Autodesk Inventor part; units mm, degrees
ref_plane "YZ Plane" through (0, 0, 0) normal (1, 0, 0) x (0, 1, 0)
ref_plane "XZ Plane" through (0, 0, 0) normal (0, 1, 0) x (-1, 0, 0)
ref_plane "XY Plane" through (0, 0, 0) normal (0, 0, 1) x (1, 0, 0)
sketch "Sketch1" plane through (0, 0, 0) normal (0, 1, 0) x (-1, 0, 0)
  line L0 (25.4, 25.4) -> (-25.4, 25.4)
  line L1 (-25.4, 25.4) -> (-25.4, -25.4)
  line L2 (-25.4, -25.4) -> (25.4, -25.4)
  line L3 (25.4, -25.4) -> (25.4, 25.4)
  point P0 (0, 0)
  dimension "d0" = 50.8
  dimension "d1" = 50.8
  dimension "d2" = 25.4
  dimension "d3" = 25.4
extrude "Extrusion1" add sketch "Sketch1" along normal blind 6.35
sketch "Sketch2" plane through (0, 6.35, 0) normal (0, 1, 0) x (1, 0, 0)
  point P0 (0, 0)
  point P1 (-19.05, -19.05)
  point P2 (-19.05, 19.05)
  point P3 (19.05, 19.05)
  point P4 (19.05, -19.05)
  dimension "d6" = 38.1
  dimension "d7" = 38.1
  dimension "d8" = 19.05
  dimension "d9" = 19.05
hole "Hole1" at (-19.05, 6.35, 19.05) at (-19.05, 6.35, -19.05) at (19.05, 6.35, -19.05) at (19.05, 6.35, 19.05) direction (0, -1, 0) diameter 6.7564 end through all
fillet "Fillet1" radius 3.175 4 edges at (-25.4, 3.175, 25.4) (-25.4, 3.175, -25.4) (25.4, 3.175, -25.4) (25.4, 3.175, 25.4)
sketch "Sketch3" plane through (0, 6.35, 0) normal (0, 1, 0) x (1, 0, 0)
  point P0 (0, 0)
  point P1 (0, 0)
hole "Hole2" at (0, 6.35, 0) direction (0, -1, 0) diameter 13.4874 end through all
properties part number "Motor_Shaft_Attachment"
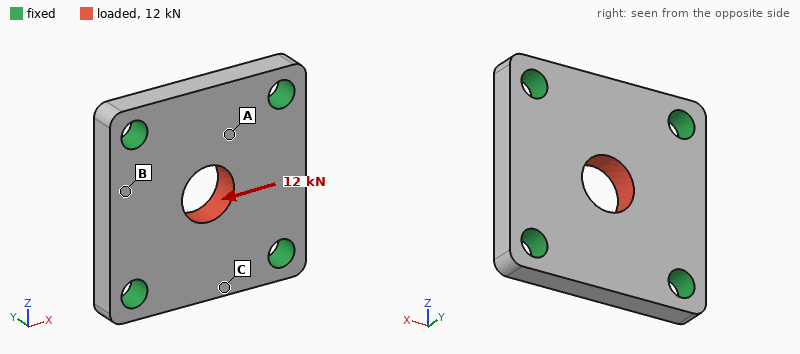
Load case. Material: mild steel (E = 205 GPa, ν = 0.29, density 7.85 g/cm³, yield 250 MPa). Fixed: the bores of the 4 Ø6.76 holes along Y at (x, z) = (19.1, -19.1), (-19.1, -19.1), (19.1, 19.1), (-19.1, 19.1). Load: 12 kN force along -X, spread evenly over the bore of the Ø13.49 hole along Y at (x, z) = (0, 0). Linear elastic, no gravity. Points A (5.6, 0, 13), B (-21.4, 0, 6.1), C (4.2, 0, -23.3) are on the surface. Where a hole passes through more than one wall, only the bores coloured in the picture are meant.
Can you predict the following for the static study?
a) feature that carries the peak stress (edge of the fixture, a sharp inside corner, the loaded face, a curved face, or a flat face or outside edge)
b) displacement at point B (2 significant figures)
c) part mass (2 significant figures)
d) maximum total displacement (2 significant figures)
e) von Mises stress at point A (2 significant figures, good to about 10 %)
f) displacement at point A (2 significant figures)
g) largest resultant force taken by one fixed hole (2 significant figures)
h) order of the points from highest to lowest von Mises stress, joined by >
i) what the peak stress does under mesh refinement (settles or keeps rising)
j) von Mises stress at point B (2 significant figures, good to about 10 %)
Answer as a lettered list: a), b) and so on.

a) edge of the fixture
b) 2.9 µm
c) 110 g
d) 5.1 µm
e) 32 MPa
f) 2.0 µm
g) 3.3 kN
h) A > B > C
i) keeps rising
j) 16 MPa
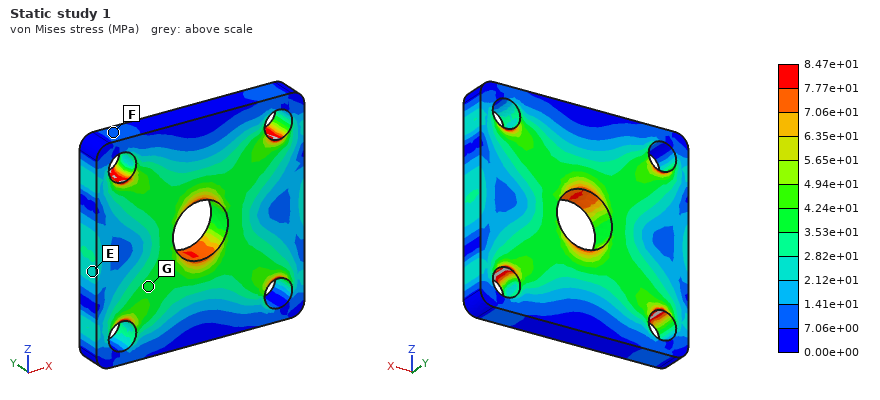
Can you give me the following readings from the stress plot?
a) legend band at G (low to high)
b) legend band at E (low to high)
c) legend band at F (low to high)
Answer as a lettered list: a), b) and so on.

a) 3.53e+01 to 4.24e+01 MPa
b) 2.12e+01 to 2.82e+01 MPa
c) 7.06e+00 to 1.41e+01 MPa
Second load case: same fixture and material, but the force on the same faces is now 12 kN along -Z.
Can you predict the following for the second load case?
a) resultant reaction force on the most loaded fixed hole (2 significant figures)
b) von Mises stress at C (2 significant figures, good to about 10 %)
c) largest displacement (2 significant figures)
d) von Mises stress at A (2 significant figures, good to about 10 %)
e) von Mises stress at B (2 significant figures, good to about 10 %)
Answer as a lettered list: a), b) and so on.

a) 3.3 kN
b) 16 MPa
c) 5.1 µm
d) 33 MPa
e) 9.9 MPa
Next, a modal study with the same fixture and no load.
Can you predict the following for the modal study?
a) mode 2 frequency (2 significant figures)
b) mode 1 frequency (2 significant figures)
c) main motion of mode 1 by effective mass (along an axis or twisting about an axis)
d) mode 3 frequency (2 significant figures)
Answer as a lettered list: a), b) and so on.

a) 25 kHz
b) 17 kHz
c) along Y
d) 25 kHz
